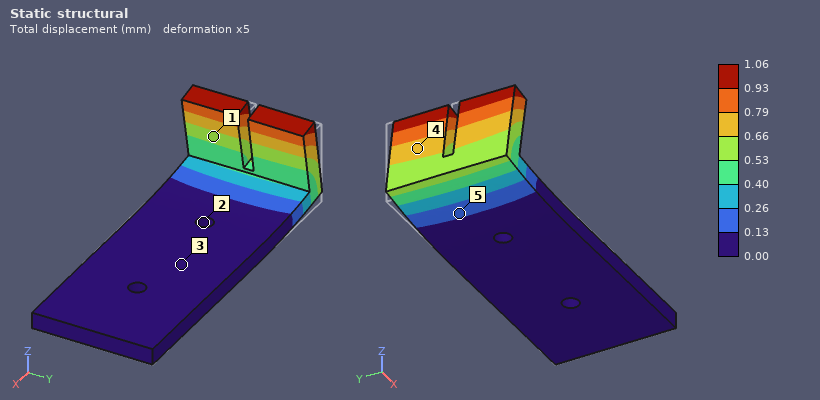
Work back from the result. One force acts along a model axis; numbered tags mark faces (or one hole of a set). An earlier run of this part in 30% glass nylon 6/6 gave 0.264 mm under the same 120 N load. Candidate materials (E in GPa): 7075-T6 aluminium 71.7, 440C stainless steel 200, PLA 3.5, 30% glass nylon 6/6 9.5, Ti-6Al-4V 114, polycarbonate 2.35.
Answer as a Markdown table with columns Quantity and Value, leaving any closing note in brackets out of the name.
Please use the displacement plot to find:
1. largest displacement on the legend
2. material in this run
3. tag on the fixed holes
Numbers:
| Quantity | Value |
|---|---|
| largest displacement on the legend | 1.06 mm |
| material in this run | polycarbonate |
| tag on the fixed holes | 2 |
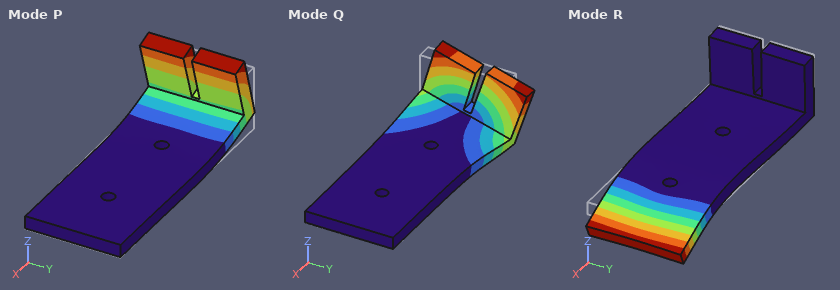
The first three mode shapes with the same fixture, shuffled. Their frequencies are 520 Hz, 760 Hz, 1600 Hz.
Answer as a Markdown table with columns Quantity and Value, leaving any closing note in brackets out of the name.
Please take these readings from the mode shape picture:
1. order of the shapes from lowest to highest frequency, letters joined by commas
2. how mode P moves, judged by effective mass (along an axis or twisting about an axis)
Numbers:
| Quantity | Value |
|---|---|
| order of the shapes from lowest to highest frequency, letters joined by commas | P, Q, R |
| how mode P moves, judged by effective mass | along Z |
